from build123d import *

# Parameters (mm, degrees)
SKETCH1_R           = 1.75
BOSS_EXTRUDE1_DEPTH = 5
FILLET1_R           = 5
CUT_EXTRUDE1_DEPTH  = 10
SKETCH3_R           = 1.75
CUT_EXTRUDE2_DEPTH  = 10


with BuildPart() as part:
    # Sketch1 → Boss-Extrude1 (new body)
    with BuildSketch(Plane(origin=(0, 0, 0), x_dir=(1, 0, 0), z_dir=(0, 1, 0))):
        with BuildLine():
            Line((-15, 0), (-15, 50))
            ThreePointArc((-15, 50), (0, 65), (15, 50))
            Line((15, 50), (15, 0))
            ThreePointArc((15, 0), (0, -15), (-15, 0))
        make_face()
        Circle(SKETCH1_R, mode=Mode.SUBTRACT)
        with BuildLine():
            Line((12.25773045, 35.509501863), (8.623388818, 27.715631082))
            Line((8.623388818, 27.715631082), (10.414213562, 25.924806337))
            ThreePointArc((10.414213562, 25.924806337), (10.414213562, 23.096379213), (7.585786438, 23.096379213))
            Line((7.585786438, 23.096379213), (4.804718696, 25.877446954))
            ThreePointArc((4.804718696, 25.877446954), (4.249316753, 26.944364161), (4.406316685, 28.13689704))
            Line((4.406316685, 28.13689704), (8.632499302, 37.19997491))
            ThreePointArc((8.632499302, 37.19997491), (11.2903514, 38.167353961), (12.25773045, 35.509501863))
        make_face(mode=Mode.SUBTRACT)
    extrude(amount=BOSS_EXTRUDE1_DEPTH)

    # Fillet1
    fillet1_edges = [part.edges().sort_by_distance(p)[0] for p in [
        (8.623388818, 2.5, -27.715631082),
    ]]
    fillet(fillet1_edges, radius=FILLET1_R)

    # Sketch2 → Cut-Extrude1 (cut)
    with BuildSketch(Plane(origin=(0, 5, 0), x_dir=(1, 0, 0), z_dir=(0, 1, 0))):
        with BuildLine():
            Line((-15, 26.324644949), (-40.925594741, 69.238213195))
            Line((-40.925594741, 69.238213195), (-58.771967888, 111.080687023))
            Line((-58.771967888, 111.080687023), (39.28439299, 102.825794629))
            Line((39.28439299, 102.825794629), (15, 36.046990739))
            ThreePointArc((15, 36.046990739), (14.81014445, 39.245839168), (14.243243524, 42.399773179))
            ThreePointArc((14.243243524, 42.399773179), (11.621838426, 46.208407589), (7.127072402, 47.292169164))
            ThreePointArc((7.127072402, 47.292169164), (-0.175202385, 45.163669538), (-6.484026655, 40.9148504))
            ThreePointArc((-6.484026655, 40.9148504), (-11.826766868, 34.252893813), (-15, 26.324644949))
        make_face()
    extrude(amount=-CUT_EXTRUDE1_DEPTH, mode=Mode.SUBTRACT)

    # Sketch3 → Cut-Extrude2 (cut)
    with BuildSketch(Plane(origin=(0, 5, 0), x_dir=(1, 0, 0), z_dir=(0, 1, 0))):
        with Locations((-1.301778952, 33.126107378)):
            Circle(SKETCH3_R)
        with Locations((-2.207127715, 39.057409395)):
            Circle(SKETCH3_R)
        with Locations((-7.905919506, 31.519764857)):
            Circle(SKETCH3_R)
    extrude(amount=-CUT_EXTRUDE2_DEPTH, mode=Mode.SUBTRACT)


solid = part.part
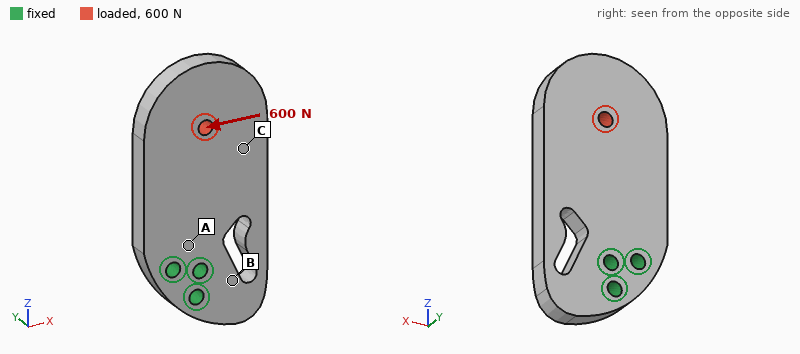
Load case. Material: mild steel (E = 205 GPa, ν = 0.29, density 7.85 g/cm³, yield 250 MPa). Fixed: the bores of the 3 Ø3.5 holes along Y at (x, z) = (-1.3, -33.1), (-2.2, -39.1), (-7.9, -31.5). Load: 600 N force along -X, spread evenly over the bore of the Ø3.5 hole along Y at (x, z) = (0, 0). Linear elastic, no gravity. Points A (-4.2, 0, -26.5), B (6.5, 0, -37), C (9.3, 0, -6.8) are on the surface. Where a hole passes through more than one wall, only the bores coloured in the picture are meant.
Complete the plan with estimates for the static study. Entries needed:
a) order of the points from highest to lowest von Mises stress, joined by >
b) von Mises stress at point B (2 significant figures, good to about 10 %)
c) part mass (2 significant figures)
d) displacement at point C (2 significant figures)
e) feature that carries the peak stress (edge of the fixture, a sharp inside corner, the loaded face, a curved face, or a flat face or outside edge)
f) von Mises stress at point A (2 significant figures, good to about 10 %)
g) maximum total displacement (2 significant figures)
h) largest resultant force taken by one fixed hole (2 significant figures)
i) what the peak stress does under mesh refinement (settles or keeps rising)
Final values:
A > B > C
20 MPa
60 g
11 µm
edge of the fixture
29 MPa
18 µm
1.5 kN
keeps rising
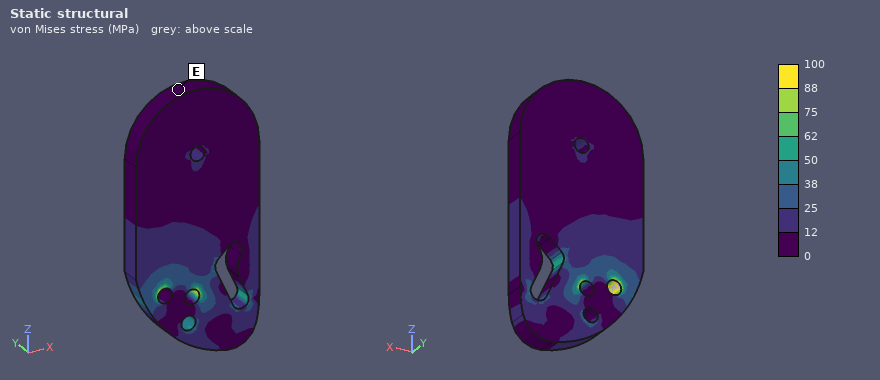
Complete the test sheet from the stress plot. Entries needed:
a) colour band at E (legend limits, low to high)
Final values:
0 to 12 MPa
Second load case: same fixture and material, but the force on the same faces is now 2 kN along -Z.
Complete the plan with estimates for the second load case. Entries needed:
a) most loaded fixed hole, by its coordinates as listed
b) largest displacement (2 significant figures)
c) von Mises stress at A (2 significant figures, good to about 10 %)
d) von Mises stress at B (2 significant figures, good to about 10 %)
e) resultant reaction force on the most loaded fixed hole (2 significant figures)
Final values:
(-1.3, -33.1)
8.5 µm
21 MPa
14 MPa
1.5 kN
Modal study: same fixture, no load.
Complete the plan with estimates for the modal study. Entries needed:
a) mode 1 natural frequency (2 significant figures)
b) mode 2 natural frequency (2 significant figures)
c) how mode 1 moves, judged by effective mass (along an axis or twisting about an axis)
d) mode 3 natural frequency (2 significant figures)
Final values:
1900 Hz
5800 Hz
along Y
5900 Hz
